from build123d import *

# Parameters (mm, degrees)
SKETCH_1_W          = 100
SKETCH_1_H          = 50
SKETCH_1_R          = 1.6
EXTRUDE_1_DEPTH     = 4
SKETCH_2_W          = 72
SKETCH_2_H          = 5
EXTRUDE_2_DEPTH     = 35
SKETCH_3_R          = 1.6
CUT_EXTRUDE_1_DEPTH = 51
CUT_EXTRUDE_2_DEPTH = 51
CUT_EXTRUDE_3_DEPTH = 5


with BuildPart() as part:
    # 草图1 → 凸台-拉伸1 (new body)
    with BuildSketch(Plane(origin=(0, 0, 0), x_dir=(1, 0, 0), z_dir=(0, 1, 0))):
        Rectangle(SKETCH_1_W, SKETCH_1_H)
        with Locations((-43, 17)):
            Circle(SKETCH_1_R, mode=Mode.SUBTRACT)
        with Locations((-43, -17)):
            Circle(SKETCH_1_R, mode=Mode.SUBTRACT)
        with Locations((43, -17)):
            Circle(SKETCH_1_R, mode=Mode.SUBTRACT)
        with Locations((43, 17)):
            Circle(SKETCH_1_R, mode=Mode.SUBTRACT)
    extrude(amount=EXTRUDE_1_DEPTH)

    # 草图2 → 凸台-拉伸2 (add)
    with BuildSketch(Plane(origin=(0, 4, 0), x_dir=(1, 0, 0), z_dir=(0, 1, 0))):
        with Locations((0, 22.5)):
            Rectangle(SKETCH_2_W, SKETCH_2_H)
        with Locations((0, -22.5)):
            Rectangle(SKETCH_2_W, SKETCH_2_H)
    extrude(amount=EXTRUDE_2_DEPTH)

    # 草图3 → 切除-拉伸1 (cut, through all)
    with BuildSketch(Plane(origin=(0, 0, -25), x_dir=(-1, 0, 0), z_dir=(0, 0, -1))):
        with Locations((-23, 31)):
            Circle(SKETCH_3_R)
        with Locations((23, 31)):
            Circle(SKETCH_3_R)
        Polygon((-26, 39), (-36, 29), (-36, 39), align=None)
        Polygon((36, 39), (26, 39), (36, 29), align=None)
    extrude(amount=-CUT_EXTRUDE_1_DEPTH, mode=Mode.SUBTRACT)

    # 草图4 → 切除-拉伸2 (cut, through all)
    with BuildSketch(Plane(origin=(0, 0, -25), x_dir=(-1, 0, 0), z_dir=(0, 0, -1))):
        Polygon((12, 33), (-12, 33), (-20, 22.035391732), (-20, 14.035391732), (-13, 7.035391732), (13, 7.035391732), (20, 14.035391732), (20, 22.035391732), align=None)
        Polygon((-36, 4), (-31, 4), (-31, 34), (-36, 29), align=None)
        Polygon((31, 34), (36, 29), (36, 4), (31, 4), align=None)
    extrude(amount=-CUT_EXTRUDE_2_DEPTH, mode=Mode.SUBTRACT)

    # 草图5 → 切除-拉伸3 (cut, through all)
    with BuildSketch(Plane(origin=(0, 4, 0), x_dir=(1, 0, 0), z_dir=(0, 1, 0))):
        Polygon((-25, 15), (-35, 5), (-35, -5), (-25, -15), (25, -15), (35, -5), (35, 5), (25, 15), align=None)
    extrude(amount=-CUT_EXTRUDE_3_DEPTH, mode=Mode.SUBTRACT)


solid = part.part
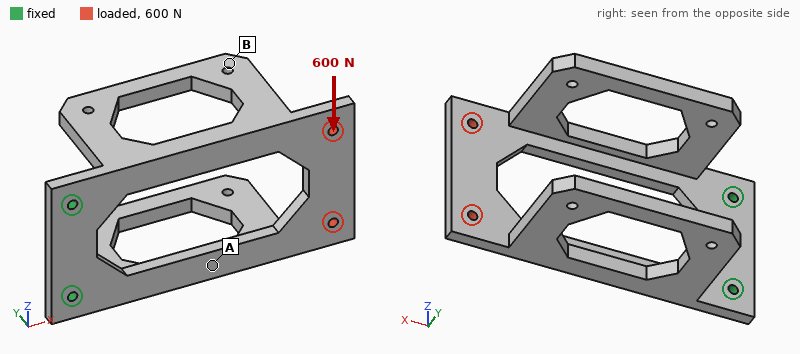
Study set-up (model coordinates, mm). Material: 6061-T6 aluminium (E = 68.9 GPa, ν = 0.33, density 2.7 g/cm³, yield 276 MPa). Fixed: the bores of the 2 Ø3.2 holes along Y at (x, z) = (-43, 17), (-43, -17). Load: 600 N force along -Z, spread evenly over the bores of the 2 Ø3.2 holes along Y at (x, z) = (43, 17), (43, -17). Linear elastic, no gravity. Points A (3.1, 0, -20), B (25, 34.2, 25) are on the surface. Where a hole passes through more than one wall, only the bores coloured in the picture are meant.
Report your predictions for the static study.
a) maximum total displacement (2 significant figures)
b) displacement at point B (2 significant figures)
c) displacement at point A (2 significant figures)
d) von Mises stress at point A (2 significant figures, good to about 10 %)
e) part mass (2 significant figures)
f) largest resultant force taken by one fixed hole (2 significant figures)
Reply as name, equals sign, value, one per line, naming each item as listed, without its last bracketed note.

maximum total displacement = 0.35 mm
displacement at point B = 0.27 mm
displacement at point A = 0.19 mm
von Mises stress at point A = 27 MPa
part mass = 66 g
largest resultant force taken by one fixed hole = 1.4 kN
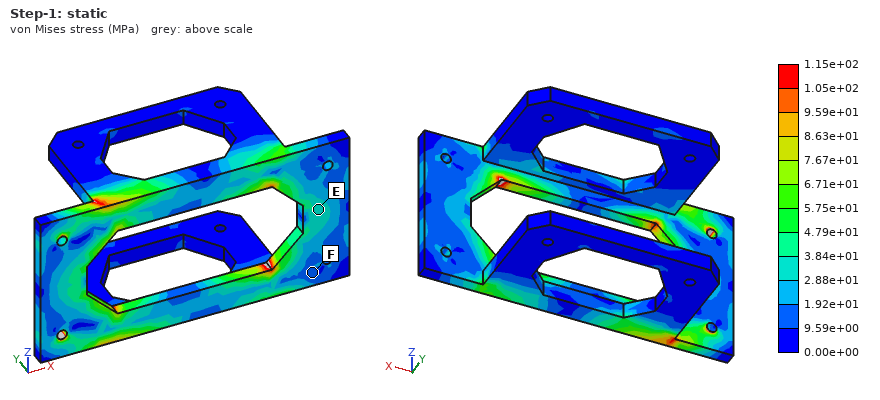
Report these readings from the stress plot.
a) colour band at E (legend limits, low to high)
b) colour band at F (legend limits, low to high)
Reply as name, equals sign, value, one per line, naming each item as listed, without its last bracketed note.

colour band at E = 2.88e+01 to 3.84e+01 MPa
colour band at F = 9.59e+00 to 1.92e+01 MPa
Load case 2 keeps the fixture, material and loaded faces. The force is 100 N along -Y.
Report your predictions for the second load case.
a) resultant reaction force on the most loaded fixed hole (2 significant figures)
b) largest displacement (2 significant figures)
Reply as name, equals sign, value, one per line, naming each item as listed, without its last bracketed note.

resultant reaction force on the most loaded fixed hole = 53 N
largest displacement = 0.99 mm
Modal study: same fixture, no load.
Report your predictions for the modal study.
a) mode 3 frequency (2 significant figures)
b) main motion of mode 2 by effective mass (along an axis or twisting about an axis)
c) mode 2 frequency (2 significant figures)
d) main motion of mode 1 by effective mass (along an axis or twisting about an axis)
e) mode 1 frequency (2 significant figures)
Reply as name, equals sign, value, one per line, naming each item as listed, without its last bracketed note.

mode 3 frequency = 1100 Hz
main motion of mode 2 by effective mass = along Z
mode 2 frequency = 680 Hz
main motion of mode 1 by effective mass = along Y
mode 1 frequency = 340 Hz
